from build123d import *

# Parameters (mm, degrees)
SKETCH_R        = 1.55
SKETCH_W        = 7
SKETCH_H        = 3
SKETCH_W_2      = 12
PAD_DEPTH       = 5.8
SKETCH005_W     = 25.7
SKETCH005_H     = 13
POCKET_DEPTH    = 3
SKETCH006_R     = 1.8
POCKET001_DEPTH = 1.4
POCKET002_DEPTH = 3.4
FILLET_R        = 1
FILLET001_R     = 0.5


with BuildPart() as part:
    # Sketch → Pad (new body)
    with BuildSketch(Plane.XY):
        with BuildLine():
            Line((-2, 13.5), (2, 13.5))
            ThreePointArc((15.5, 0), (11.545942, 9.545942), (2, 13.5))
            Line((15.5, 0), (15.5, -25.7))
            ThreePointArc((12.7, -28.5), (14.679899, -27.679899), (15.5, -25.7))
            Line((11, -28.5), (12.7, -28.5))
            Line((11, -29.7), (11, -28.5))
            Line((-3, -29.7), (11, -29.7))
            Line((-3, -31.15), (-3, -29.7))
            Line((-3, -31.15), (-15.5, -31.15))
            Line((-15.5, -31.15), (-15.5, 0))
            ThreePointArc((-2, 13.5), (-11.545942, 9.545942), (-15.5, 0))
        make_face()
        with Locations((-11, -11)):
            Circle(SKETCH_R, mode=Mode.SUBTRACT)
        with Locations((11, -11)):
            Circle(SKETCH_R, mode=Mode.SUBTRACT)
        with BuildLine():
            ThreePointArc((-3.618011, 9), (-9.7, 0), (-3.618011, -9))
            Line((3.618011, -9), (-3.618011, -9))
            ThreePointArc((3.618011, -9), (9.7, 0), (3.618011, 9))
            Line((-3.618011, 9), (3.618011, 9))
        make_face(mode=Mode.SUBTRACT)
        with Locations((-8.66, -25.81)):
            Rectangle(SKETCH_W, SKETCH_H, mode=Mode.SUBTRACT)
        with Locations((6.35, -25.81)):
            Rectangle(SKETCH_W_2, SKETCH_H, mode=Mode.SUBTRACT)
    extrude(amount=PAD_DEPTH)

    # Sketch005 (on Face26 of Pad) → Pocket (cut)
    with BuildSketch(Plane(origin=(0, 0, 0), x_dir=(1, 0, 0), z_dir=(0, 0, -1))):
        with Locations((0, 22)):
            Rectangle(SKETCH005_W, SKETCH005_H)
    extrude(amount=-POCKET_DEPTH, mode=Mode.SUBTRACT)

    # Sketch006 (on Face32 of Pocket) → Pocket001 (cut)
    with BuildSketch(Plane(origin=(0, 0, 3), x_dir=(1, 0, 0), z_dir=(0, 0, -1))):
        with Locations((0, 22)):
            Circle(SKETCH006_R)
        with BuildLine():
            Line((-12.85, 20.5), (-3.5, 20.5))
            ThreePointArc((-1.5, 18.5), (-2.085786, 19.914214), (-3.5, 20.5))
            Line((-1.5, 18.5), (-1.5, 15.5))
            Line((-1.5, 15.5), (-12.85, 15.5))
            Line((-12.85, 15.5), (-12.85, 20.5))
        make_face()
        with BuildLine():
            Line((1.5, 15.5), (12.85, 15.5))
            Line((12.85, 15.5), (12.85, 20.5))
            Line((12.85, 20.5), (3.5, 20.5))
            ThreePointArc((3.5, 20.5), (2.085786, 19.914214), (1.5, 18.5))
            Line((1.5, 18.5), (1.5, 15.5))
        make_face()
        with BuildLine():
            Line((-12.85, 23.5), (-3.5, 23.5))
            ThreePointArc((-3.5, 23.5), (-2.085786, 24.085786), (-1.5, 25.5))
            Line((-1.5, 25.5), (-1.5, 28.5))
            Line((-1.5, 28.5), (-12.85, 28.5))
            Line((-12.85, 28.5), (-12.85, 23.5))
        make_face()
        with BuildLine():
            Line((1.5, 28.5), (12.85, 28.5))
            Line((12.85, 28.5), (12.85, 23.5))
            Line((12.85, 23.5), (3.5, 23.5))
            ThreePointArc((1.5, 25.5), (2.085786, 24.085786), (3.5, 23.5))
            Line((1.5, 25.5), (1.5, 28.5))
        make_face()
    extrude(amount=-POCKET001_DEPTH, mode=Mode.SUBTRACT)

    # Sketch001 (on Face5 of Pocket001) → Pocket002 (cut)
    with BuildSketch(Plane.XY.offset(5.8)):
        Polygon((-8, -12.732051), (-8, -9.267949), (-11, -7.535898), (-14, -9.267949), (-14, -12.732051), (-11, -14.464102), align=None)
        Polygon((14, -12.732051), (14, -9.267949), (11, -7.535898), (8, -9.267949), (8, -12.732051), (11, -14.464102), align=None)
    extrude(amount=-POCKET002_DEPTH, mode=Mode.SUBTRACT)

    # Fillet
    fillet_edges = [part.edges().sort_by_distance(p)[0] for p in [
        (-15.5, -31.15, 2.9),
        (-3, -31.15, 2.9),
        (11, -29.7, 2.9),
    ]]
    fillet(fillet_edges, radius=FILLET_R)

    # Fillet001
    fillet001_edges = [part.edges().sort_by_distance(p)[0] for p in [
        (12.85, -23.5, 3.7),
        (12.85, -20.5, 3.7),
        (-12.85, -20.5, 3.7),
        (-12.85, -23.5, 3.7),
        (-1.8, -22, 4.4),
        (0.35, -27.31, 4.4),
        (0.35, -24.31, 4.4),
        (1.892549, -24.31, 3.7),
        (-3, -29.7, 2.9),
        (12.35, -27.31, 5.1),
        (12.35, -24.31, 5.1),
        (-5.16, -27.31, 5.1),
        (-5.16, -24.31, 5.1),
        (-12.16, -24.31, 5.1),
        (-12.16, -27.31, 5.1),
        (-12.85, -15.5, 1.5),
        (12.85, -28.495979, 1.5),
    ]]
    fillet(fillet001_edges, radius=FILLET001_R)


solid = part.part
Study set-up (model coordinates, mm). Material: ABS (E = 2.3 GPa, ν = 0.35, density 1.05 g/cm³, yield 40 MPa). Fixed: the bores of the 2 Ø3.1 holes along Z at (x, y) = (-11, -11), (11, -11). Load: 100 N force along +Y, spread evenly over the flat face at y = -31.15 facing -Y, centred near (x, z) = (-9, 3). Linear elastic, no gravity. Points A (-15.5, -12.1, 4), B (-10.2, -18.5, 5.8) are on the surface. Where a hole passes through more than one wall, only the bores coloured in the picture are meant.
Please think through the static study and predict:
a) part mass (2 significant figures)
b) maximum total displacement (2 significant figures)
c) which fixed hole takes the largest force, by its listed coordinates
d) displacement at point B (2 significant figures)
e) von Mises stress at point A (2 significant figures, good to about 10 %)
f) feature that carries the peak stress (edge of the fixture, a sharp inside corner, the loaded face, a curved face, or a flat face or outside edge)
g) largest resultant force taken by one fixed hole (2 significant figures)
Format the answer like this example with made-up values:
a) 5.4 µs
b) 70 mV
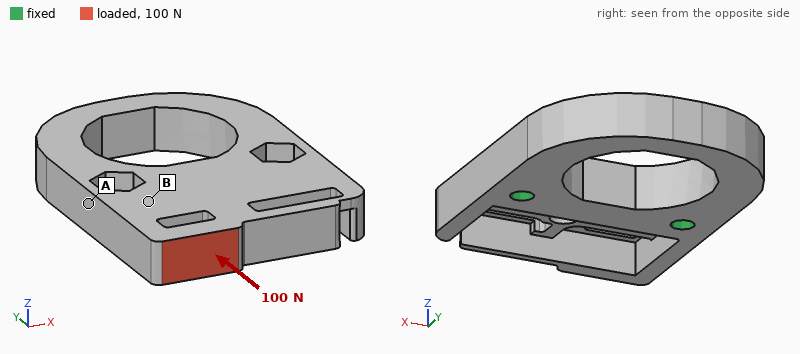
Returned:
a) 4.2 g
b) 0.17 mm
c) (-11, -11)
d) 0.028 mm
e) 2.9 MPa
f) a curved face
g) 88 N
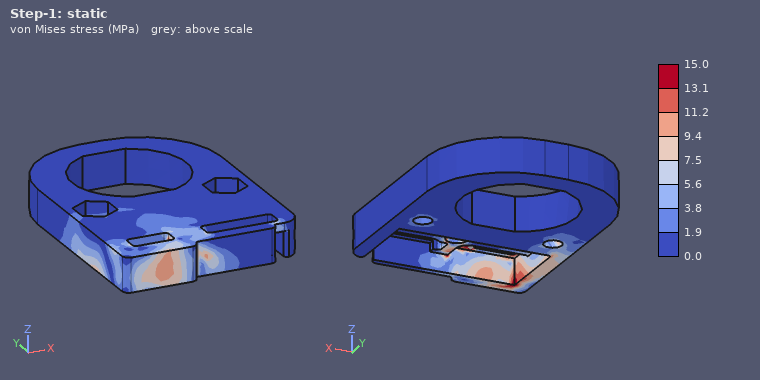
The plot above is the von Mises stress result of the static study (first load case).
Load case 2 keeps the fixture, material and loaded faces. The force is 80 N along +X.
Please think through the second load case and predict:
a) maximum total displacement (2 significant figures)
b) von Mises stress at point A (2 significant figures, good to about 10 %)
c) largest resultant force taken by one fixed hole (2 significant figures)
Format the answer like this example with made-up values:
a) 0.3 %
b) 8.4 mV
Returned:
a) 0.35 mm
b) 6.7 MPa
c) 77 N
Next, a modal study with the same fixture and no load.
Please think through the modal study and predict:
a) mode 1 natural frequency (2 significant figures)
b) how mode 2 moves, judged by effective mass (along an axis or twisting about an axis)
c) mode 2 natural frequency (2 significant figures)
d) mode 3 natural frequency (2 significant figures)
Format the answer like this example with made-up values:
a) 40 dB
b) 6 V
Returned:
a) 1300 Hz
b) along Z
c) 2100 Hz
d) 2900 Hz
